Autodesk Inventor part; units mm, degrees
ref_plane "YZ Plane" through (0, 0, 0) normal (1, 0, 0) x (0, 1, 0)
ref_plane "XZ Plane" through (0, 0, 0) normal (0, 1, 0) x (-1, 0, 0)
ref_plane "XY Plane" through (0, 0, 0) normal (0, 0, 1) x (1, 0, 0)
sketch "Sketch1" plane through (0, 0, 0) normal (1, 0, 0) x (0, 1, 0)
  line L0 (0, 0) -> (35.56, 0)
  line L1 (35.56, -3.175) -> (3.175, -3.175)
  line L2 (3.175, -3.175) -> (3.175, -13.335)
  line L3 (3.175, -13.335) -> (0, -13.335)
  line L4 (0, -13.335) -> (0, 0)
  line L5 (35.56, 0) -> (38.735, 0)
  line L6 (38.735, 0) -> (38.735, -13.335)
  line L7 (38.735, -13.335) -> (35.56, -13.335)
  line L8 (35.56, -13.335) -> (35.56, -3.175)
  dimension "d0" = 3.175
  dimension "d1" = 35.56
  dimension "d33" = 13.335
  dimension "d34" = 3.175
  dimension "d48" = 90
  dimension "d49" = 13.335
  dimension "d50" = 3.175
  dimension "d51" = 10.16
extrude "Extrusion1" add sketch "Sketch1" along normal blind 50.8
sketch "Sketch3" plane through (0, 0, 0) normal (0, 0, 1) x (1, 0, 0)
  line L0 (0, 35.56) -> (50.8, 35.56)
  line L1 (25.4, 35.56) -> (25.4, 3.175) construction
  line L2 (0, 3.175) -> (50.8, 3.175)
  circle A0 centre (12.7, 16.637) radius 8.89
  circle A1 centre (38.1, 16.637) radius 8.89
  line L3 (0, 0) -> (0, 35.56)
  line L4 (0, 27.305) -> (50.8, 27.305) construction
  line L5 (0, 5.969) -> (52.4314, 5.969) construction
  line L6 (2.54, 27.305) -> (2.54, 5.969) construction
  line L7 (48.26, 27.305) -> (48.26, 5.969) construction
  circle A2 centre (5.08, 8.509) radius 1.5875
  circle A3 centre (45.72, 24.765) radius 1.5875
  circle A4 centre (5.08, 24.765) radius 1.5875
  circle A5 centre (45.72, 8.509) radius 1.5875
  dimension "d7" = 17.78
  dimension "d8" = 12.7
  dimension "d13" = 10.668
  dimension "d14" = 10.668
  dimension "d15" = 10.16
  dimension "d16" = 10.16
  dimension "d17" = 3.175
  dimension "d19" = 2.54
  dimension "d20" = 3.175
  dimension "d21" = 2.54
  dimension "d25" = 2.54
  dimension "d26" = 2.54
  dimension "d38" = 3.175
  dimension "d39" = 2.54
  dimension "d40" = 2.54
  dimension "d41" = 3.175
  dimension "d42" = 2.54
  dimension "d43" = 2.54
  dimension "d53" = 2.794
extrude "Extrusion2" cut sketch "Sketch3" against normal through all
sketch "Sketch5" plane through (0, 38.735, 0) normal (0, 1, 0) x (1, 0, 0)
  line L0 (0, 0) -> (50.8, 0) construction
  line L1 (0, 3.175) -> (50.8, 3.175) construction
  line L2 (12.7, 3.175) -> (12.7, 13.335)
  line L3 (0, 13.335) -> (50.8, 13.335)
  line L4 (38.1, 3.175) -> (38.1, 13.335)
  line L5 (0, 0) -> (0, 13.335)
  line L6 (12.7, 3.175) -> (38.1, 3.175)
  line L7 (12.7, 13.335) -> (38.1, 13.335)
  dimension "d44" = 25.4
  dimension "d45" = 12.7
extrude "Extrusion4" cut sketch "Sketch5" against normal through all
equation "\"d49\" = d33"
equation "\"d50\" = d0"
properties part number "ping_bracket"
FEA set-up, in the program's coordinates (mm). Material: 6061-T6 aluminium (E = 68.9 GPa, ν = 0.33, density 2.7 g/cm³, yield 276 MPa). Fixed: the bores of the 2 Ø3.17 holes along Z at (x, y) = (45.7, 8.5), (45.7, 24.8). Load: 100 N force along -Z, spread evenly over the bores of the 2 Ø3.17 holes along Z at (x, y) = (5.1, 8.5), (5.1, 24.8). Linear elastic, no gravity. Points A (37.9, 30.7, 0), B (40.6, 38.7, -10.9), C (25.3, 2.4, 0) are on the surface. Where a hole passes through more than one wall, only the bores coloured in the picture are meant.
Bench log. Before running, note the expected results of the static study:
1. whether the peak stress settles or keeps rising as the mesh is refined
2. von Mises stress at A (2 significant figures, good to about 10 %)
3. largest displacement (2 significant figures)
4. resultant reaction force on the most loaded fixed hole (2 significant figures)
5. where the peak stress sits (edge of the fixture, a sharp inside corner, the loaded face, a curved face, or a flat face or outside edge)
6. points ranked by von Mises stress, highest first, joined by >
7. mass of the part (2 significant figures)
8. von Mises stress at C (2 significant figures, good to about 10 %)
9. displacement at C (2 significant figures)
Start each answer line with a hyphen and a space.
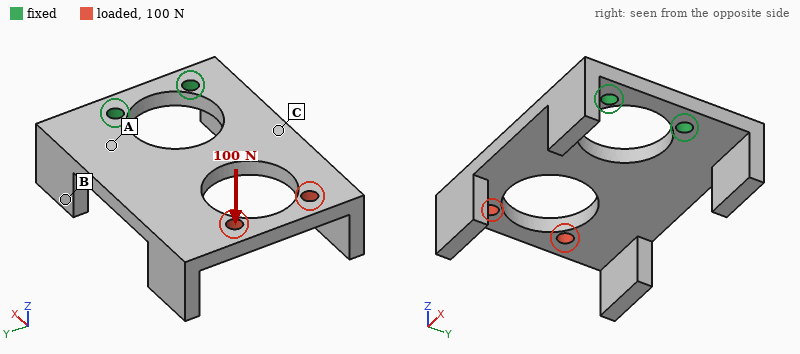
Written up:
- keeps rising
- 76 MPa
- 0.67 mm
- 54 N
- edge of the fixture
- A > C > B
- 17 g
- 46 MPa
- 0.17 mm
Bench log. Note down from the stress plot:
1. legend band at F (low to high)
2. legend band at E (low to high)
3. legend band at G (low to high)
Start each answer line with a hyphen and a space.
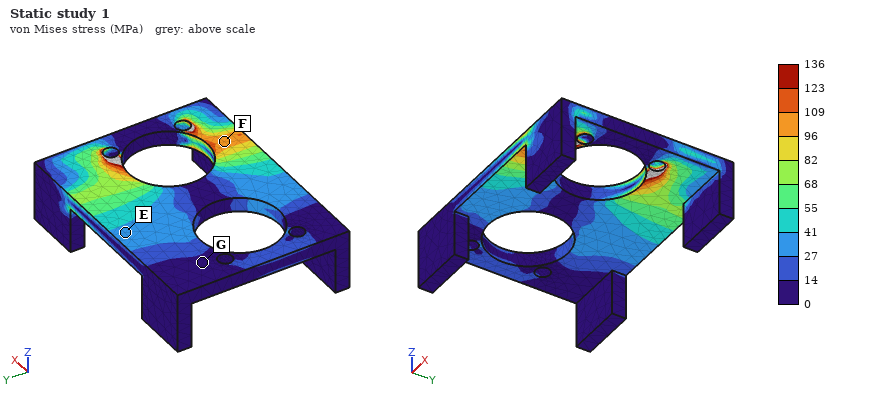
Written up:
- 96 to 109 MPa
- 27 to 41 MPa
- 0 to 14 MPa
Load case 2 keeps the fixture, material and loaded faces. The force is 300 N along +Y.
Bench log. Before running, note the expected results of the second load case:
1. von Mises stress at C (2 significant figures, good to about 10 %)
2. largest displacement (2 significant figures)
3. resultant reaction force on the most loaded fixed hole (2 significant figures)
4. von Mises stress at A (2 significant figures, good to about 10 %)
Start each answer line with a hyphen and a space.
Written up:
- 11 MPa
- 75 µm
- 480 N
- 12 MPa
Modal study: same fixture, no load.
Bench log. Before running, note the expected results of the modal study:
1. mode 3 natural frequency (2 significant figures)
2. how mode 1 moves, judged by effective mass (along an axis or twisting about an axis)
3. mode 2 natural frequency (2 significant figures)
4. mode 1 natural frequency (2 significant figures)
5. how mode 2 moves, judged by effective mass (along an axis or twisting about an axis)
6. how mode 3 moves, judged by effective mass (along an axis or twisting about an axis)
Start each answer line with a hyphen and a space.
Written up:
- 4000 Hz
- along Z
- 1900 Hz
- 880 Hz
- twisting about X
- along Y
